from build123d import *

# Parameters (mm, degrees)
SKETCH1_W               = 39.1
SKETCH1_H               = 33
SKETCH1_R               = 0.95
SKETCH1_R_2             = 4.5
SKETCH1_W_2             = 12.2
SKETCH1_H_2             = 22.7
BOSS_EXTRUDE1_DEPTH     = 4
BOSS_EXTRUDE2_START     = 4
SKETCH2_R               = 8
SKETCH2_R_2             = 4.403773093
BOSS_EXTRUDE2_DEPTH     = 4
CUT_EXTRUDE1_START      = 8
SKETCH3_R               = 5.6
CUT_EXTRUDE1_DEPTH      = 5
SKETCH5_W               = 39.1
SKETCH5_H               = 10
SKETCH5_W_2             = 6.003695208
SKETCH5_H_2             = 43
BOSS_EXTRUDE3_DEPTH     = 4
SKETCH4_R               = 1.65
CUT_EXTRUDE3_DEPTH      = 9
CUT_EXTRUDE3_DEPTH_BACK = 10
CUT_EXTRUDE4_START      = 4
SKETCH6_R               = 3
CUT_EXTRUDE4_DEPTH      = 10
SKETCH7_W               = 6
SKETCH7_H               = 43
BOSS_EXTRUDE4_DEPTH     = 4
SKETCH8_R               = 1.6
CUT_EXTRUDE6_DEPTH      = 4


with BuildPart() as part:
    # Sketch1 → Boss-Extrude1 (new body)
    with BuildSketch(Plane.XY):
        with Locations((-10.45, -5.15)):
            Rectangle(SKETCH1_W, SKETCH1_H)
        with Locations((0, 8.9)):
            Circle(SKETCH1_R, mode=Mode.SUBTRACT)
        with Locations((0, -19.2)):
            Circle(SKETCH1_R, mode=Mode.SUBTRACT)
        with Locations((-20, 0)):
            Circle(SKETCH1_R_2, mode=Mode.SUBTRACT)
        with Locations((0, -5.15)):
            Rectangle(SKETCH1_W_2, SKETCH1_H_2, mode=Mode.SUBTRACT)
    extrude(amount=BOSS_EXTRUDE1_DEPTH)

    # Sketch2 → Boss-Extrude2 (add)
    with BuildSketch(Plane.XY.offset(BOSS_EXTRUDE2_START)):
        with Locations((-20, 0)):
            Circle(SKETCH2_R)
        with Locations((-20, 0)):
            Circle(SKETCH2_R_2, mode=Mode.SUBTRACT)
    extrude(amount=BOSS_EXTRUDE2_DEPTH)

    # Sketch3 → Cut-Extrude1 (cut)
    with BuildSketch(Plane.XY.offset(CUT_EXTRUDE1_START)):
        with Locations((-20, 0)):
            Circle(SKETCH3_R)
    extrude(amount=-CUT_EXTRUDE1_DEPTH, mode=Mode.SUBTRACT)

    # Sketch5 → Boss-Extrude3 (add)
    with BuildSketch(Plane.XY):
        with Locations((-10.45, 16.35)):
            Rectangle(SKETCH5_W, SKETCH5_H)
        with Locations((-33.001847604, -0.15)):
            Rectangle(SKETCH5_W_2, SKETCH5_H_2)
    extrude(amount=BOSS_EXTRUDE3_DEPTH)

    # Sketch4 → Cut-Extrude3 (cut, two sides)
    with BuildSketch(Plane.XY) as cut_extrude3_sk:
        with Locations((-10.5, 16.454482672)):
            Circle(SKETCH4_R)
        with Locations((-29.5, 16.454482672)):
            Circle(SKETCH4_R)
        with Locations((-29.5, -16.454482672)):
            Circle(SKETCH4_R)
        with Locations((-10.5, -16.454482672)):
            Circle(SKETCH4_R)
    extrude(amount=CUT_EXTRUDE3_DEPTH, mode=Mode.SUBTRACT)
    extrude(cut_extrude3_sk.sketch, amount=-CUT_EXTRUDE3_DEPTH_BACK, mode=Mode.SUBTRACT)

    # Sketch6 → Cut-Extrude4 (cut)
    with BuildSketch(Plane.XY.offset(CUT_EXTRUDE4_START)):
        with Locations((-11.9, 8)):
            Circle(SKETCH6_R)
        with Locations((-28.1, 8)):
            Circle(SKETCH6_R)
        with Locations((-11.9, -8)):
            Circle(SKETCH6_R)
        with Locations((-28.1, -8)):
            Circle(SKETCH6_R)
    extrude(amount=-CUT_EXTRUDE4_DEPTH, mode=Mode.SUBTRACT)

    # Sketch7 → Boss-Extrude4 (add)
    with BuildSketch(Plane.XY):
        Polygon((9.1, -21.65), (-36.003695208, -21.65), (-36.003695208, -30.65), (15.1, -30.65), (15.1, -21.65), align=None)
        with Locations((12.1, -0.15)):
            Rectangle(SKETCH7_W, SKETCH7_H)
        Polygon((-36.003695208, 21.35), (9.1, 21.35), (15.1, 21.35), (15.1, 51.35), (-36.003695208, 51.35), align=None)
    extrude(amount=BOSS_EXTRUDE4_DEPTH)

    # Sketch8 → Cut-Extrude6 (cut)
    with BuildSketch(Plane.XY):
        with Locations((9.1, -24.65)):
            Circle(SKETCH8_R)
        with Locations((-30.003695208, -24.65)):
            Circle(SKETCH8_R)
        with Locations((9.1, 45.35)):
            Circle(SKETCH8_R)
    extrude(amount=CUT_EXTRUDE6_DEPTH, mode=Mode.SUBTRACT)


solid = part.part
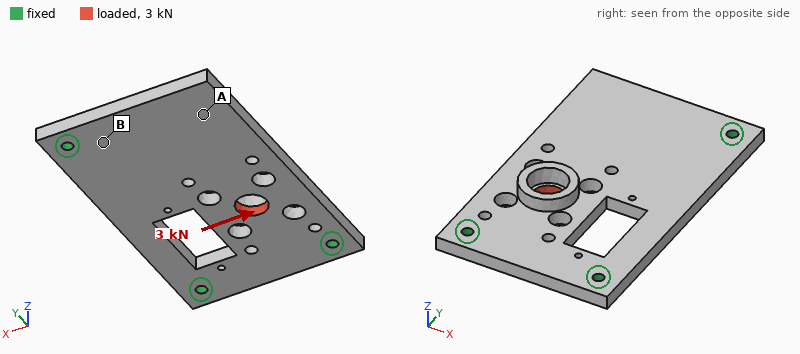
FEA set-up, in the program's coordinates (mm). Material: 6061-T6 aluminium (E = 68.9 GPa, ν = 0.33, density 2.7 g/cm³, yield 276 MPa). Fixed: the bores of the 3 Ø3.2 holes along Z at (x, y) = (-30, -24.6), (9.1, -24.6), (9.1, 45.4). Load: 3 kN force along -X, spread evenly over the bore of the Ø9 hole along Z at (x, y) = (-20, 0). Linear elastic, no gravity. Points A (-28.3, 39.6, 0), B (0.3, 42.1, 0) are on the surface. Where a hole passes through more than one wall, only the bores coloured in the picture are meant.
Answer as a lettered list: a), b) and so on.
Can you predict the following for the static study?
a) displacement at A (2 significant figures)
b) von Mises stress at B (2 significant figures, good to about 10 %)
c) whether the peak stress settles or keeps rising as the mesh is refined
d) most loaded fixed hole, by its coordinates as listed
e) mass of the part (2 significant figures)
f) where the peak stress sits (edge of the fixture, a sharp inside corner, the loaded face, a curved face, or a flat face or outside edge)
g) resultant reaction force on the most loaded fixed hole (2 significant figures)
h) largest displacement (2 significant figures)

a) 24 µm
b) 21 MPa
c) keeps rising
d) (9.1, 45.4)
e) 41 g
f) a sharp inside corner
g) 1.2 kN
h) 40 µm
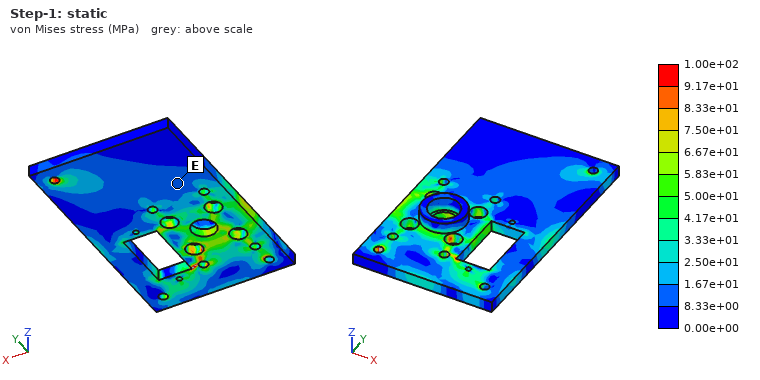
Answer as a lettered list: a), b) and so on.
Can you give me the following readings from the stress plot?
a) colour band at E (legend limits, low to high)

a) 8.33e+00 to 1.67e+01 MPa
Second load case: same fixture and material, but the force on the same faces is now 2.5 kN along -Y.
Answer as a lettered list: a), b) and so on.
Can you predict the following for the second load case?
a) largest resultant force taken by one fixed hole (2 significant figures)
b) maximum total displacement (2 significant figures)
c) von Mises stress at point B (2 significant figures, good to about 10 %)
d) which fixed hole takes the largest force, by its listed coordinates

a) 1.4 kN
b) 29 µm
c) 6.2 MPa
d) (-30, -24.6)
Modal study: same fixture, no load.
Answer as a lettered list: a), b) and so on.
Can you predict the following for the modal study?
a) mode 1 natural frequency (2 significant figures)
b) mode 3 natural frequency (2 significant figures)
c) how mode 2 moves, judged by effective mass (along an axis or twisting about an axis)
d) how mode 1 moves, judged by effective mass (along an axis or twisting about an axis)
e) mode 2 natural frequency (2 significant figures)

a) 1800 Hz
b) 5500 Hz
c) along Z
d) along Z
e) 3700 Hz
